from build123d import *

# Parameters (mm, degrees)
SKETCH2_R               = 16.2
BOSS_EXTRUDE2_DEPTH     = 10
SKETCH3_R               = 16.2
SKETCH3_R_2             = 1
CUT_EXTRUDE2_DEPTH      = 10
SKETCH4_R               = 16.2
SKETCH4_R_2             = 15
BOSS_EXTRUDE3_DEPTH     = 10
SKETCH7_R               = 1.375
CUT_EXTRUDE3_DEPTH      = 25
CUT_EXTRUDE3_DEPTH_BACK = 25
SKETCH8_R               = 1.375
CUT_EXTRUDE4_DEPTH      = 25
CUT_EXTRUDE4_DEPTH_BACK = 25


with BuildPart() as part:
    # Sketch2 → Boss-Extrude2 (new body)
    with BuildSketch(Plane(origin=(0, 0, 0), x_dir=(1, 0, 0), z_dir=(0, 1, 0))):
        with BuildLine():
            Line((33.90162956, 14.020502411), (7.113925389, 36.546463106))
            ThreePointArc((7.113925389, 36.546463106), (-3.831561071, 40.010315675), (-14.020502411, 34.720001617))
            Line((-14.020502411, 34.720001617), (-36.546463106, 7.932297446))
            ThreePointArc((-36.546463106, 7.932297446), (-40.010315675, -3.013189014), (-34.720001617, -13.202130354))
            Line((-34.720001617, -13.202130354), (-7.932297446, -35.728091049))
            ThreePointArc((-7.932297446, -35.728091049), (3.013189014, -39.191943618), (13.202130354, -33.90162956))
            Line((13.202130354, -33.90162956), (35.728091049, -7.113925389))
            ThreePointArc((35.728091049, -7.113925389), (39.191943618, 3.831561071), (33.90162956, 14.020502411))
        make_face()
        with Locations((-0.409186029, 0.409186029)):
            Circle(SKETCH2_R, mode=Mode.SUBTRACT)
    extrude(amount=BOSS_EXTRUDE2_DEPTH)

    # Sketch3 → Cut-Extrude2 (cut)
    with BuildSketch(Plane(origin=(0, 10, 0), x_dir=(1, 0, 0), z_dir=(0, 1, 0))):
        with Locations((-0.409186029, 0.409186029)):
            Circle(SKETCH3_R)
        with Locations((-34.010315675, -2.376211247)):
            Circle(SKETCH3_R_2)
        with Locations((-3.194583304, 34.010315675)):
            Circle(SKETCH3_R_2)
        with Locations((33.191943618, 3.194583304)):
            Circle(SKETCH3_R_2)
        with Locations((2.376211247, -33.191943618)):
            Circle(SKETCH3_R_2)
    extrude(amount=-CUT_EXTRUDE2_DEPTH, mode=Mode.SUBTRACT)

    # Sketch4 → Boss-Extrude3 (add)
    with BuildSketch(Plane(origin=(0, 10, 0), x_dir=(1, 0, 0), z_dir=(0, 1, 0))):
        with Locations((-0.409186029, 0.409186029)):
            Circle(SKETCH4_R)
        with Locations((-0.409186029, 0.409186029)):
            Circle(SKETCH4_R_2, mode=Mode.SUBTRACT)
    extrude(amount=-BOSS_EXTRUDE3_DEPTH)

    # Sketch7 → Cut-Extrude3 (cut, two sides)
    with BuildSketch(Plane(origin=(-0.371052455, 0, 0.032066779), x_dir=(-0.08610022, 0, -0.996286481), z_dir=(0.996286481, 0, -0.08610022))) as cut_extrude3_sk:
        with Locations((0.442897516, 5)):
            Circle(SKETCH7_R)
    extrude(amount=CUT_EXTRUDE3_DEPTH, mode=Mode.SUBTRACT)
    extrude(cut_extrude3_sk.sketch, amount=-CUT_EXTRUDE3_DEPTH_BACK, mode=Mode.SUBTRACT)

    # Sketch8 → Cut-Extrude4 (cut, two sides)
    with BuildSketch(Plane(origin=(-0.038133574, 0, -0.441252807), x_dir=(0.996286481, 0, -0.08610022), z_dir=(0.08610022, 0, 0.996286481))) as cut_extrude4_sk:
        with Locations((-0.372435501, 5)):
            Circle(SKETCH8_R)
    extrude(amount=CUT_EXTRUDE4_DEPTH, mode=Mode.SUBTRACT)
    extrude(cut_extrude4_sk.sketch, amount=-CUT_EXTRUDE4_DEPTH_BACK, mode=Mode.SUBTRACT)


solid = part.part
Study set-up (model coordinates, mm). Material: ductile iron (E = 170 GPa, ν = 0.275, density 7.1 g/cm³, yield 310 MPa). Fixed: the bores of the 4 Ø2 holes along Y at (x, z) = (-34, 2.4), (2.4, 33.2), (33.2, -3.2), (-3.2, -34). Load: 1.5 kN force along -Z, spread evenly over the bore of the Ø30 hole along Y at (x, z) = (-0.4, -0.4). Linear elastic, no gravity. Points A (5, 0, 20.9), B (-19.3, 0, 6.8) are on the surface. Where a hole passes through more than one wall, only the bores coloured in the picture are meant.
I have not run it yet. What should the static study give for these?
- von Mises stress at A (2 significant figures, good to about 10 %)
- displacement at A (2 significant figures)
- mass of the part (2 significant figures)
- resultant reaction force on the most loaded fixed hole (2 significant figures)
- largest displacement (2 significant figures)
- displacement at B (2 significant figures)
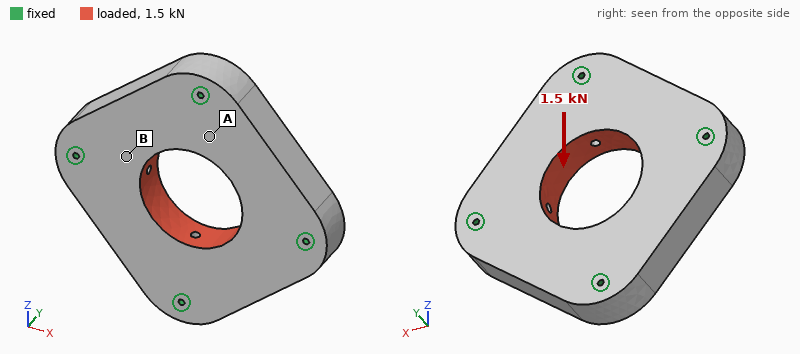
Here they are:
3.2 MPa
0.28 µm
230 g
470 N
0.56 µm
0.43 µm
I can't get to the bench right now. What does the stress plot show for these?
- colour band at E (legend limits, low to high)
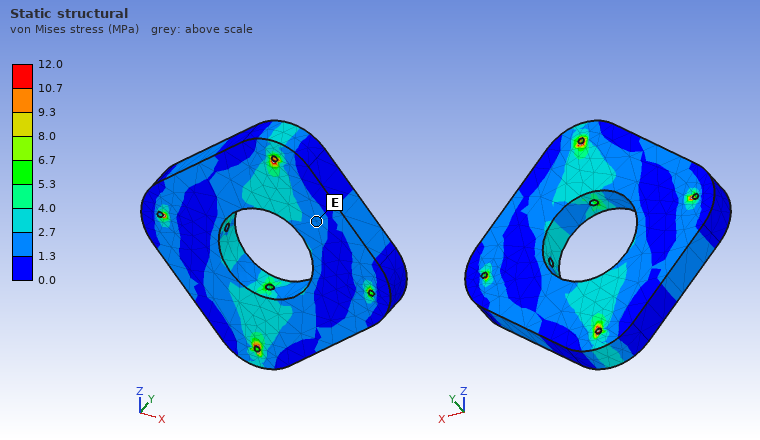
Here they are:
1.3 to 2.7 MPa
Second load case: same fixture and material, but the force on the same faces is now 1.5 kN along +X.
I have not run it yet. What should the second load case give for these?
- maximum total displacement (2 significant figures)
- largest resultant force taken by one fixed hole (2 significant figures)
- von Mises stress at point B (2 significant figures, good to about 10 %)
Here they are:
0.56 µm
470 N
3.1 MPa
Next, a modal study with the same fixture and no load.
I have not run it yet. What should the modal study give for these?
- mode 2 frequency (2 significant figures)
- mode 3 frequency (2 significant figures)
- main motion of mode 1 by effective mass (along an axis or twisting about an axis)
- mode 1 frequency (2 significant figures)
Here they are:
15 kHz
15 kHz
along Y
13 kHz
